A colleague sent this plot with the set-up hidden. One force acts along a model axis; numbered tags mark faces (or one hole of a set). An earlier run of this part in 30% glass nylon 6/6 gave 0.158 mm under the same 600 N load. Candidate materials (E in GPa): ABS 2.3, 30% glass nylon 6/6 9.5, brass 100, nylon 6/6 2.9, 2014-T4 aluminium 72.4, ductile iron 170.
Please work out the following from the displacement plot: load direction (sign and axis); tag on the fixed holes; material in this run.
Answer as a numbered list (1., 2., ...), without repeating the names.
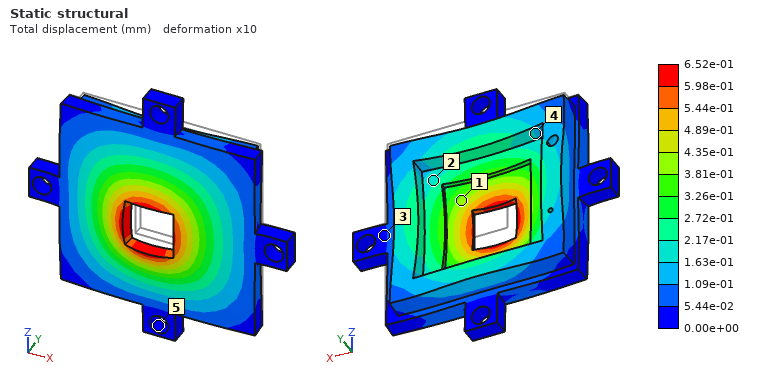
1. -Y
2. 5
3. ABS
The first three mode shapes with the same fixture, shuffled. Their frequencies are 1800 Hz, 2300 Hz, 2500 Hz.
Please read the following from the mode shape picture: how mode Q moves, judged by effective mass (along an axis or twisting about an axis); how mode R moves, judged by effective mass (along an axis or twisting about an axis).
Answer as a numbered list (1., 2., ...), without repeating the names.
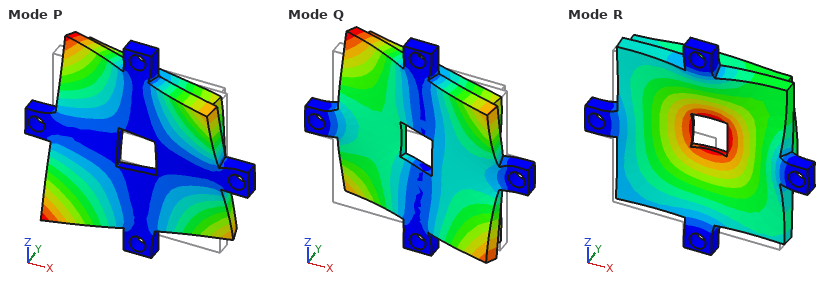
1. twisting about Z
2. along Y
